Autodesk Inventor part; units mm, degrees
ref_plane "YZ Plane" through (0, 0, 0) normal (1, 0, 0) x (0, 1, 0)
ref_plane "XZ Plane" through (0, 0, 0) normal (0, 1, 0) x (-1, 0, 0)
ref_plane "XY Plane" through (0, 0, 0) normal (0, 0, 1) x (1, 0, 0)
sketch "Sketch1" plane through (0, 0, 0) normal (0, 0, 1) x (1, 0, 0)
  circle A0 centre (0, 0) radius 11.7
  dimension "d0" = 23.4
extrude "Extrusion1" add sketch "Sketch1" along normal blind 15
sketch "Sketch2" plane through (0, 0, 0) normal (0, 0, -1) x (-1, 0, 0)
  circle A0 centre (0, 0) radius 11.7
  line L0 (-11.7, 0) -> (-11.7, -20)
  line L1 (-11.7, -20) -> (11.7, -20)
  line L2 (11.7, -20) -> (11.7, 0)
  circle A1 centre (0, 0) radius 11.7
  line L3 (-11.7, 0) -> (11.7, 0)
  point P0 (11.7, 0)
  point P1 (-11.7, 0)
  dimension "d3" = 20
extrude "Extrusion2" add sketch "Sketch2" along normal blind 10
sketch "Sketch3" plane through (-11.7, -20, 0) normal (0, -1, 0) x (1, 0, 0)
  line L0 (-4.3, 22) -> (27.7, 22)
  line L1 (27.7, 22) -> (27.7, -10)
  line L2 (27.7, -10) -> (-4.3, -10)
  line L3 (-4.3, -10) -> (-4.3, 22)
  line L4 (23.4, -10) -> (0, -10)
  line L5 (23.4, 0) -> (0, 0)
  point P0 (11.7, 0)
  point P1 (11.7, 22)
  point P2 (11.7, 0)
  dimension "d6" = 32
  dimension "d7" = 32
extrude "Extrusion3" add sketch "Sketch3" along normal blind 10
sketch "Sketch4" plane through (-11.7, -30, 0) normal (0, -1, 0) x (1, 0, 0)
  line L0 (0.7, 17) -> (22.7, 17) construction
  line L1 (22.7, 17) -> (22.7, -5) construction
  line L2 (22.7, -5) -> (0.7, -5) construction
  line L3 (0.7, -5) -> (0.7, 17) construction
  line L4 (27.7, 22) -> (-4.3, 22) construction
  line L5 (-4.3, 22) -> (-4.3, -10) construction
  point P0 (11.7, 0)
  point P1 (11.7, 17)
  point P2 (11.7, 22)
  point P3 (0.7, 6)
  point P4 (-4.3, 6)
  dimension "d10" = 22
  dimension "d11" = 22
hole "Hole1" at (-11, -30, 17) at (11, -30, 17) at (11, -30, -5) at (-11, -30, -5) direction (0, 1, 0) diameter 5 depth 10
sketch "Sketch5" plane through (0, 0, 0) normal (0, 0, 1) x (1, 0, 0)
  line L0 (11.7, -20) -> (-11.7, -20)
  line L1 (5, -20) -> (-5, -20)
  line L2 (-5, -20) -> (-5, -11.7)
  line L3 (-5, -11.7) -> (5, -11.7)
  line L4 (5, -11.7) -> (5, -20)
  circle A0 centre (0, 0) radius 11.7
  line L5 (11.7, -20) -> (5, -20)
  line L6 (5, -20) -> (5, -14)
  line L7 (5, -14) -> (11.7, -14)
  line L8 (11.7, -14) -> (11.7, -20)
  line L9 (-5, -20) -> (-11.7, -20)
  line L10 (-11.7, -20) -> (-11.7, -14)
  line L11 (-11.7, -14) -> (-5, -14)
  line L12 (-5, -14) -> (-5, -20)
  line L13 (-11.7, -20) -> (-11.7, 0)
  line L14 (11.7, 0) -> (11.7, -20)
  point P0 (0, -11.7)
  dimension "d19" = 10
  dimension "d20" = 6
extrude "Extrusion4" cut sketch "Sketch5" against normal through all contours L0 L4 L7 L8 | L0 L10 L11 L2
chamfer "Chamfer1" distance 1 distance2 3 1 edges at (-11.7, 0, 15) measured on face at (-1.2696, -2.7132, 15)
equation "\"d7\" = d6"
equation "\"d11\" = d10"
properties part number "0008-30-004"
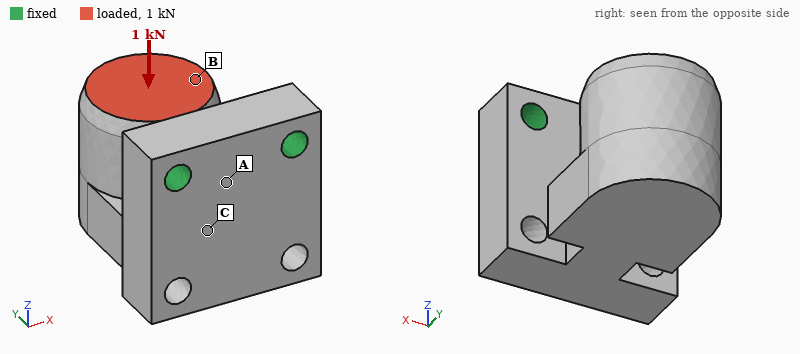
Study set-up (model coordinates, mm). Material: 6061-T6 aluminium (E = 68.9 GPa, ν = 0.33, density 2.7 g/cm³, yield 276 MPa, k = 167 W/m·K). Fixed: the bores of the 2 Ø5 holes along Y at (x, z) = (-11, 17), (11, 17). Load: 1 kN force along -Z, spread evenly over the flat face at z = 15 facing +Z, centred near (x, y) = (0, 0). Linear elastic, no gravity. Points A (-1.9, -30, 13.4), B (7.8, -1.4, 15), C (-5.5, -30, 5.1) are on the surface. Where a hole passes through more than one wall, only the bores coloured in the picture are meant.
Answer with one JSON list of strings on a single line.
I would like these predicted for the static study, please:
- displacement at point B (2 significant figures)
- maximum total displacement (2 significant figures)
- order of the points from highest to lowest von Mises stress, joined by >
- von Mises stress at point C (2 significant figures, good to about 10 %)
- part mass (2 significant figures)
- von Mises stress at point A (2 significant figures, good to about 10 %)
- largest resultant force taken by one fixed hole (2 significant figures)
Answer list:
["0.17 mm", "0.24 mm", "C > A > B", "43 MPa", "59 g", "24 MPa", "540 N"]
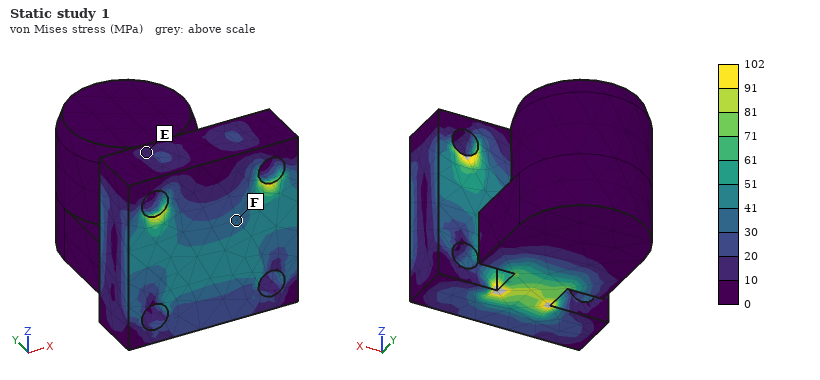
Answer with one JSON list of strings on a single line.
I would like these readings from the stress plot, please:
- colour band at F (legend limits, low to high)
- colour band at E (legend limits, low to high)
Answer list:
["30 to 41 MPa", "10 to 20 MPa"]
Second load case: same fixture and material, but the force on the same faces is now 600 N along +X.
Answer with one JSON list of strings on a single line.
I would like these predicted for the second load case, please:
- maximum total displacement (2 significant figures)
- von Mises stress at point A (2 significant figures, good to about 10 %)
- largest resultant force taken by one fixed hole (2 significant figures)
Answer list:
["0.17 mm", "8.9 MPa", "660 N"]
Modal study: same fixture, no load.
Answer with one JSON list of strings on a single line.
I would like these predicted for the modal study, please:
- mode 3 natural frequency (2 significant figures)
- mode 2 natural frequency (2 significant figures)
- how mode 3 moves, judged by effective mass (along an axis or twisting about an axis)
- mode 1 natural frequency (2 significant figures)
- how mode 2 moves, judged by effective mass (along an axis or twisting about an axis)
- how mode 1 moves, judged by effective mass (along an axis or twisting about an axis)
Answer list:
["5400 Hz", "2400 Hz", "along Y", "2200 Hz", "along X", "along Z"]
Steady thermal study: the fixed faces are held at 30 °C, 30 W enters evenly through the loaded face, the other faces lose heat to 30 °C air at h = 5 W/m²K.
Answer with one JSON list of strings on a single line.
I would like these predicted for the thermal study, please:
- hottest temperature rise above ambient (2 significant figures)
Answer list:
["45 K"]
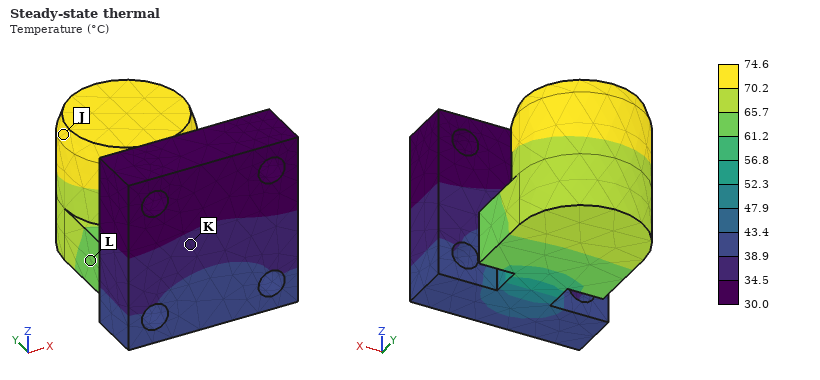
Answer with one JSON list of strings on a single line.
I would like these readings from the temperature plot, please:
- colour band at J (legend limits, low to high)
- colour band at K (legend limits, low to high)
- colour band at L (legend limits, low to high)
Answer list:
["70.2 to 74.6 °C", "34.5 to 38.9 °C", "61.2 to 65.7 °C"]
